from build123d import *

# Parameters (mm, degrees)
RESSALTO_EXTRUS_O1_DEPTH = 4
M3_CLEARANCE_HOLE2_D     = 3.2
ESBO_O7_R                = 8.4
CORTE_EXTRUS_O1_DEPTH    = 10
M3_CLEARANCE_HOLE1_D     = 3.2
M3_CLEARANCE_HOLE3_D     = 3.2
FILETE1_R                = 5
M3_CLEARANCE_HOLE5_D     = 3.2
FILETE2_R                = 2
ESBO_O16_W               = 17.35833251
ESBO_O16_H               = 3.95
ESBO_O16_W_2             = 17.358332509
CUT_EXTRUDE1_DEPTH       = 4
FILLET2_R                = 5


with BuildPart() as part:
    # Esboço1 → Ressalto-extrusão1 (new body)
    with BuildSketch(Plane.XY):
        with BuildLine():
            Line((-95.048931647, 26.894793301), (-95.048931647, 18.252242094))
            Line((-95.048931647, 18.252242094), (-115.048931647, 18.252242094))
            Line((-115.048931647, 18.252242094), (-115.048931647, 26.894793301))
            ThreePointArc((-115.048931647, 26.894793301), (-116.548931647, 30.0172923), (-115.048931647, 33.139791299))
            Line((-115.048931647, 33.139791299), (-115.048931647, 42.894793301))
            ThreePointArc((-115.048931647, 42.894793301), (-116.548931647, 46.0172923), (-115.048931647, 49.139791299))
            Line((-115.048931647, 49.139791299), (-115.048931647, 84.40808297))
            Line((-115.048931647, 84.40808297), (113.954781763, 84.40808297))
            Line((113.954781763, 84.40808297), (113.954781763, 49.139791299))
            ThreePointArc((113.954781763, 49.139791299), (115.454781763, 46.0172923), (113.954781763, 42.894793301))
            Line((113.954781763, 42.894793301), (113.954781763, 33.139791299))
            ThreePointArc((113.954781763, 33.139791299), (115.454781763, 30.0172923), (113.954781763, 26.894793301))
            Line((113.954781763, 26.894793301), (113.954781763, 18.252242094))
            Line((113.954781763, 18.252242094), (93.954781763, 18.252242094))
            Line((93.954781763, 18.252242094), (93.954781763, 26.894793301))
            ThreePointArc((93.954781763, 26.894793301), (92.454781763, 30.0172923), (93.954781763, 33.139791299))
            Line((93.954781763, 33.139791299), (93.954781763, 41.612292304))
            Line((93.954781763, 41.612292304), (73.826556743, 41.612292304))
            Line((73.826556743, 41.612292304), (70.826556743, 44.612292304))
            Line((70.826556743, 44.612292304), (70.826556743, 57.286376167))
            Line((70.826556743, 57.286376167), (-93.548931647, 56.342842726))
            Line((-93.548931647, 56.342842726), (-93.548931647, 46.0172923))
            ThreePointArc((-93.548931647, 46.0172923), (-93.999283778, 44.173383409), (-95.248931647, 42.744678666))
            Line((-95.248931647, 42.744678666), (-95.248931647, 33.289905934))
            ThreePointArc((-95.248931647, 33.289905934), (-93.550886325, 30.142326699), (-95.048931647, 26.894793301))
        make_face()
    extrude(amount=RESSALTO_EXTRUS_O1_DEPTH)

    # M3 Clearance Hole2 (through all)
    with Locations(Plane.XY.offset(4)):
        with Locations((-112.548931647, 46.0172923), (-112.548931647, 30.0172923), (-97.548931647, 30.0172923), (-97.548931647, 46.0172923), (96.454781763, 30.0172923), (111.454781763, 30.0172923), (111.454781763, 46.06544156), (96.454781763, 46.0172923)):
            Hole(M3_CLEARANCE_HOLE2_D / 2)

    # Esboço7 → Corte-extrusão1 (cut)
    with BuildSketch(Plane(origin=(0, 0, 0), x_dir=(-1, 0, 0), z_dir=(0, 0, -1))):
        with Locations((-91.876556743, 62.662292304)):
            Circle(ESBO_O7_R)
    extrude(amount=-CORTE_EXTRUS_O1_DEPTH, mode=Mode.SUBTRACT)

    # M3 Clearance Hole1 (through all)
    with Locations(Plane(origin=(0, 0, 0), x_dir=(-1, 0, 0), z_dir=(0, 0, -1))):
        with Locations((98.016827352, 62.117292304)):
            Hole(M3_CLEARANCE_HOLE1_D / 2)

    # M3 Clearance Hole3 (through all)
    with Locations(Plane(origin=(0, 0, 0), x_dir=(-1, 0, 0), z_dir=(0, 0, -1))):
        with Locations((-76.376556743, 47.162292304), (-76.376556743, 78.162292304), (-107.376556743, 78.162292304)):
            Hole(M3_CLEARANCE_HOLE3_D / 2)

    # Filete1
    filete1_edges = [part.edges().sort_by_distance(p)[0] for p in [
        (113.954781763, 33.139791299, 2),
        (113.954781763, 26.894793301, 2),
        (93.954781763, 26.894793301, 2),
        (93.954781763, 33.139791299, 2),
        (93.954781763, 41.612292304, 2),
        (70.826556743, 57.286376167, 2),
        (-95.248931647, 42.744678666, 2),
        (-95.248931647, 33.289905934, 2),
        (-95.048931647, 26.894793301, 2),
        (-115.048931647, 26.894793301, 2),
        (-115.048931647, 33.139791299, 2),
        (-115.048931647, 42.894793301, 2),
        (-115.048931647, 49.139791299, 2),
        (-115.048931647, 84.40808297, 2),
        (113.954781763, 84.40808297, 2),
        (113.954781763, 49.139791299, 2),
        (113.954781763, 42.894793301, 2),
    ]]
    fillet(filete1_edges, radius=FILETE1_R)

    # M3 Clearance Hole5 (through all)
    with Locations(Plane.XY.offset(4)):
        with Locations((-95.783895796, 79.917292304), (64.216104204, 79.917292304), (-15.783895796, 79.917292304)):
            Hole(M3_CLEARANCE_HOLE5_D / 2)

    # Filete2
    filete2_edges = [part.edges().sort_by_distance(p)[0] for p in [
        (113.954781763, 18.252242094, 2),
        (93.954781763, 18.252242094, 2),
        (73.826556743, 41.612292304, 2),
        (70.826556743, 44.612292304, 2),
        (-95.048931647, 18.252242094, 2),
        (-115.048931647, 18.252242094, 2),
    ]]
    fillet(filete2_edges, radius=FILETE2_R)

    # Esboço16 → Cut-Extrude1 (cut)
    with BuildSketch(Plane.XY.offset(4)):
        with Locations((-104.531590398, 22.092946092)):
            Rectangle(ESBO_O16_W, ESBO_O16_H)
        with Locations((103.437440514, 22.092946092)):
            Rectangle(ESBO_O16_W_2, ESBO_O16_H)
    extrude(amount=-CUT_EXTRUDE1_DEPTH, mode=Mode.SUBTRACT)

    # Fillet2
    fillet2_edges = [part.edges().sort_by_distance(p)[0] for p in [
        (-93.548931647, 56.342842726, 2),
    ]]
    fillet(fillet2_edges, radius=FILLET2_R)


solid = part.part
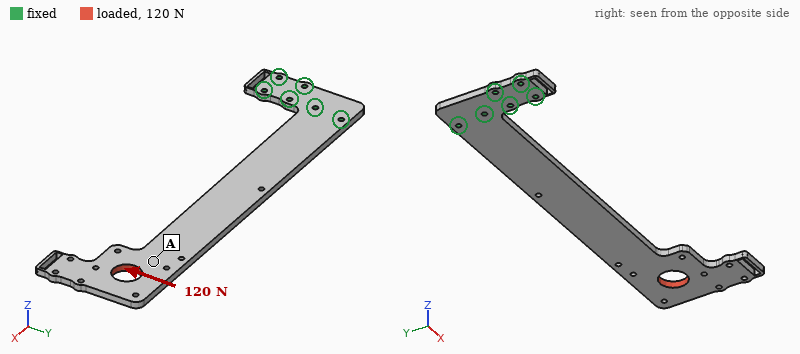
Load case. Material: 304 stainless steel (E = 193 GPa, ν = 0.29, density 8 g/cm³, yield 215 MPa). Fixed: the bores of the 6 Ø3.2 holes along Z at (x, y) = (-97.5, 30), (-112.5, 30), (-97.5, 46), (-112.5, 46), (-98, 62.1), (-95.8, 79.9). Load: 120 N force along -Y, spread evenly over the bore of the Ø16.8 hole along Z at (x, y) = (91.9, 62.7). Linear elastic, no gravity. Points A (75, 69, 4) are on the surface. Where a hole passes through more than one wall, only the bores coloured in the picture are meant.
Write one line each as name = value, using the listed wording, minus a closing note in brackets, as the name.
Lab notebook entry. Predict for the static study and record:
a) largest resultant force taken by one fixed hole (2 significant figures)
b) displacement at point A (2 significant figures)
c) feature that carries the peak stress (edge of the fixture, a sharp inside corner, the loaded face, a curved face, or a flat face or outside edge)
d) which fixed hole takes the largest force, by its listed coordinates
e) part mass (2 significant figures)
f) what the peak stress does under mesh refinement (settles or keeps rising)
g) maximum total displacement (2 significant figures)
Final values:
largest resultant force taken by one fixed hole = 1.0 kN
displacement at point A = 0.17 mm
feature that carries the peak stress = edge of the fixture
which fixed hole takes the largest force, by its listed coordinates = (-95.8, 79.9)
part mass = 250 g
what the peak stress does under mesh refinement = keeps rising
maximum total displacement = 0.25 mm
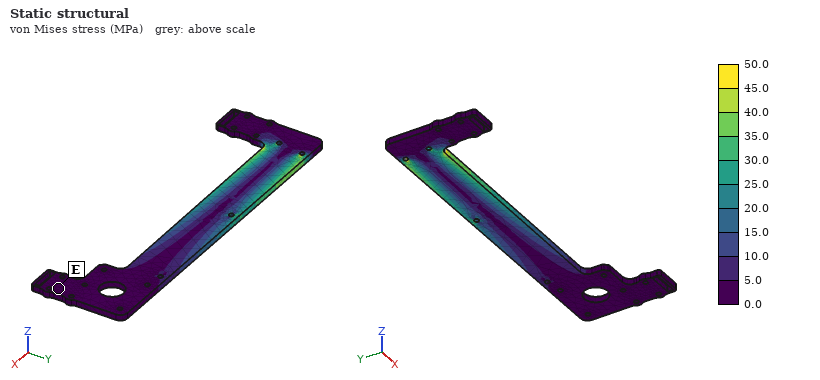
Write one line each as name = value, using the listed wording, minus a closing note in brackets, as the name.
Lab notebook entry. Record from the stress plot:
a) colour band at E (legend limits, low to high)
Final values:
colour band at E = 0.0 to 5.0 MPa
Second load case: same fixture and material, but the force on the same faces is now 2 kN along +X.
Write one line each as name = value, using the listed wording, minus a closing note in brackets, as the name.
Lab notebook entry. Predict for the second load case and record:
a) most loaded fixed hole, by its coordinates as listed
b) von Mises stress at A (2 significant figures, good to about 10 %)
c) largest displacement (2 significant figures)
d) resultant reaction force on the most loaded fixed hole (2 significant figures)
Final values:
most loaded fixed hole, by its coordinates as listed = (-98, 62.1)
von Mises stress at A = 23 MPa
largest displacement = 0.28 mm
resultant reaction force on the most loaded fixed hole = 1.4 kN
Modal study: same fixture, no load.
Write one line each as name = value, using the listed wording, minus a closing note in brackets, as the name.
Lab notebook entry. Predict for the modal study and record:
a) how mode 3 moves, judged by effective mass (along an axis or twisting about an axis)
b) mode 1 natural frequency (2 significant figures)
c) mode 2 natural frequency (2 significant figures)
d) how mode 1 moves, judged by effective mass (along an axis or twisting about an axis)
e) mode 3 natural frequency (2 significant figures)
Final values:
how mode 3 moves, judged by effective mass = along Y
mode 1 natural frequency = 60 Hz
mode 2 natural frequency = 380 Hz
how mode 1 moves, judged by effective mass = along Z
mode 3 natural frequency = 410 Hz
